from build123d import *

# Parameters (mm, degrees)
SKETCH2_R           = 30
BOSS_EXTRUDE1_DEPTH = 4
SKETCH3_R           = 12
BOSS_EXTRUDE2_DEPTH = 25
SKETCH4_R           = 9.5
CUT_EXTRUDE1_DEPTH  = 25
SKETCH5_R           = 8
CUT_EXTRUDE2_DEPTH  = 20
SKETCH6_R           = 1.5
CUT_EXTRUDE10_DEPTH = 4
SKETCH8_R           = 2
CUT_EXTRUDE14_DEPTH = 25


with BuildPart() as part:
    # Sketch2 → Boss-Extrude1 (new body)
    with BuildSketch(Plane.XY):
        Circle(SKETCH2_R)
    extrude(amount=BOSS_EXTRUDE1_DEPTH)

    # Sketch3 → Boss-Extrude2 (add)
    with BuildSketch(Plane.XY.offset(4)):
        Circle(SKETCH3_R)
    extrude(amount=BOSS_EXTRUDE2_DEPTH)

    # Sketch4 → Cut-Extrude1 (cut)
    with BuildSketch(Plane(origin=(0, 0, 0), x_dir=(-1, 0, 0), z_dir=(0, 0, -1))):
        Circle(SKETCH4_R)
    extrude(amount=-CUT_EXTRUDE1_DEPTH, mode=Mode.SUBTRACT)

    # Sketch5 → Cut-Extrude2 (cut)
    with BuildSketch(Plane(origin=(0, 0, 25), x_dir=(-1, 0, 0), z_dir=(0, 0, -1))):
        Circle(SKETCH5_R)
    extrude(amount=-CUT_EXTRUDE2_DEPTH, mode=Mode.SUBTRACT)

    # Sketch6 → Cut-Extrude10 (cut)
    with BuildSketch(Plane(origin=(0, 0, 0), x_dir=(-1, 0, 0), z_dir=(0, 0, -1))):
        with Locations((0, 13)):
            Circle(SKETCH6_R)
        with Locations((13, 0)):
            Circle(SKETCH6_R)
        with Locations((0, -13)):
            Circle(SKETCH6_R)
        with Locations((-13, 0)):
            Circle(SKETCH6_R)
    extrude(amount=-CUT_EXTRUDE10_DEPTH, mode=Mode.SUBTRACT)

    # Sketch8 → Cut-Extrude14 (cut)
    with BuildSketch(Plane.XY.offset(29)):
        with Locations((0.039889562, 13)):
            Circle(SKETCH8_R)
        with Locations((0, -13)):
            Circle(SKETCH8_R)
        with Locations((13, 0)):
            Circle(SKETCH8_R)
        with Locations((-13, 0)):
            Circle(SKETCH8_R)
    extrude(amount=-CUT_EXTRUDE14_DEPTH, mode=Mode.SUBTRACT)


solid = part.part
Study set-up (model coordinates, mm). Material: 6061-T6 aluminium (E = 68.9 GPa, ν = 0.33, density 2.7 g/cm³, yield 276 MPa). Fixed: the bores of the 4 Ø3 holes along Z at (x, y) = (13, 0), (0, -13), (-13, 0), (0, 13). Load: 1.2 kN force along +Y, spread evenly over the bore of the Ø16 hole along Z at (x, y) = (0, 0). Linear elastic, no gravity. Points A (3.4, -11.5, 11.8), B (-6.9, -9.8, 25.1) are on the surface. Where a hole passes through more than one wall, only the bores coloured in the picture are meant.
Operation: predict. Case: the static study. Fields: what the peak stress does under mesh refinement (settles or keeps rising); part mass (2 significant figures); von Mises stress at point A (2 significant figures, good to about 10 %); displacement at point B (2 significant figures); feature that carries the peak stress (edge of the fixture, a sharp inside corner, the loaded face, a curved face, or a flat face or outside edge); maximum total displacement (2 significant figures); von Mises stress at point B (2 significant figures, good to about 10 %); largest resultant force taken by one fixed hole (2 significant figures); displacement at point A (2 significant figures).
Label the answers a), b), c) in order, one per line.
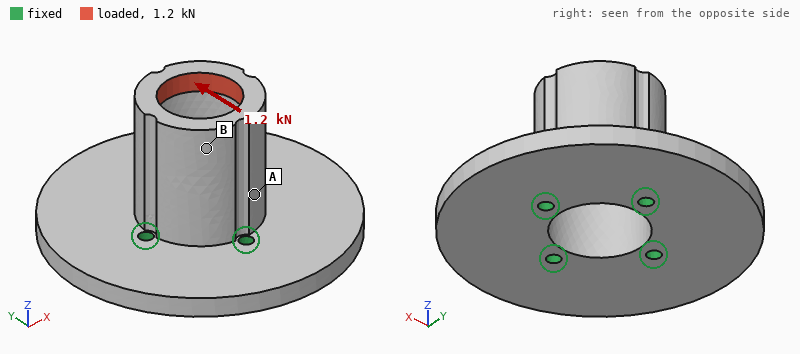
a) keeps rising
b) 39 g
c) 23 MPa
d) 29 µm
e) edge of the fixture
f) 36 µm
g) 8.4 MPa
h) 1.2 kN
i) 12 µm
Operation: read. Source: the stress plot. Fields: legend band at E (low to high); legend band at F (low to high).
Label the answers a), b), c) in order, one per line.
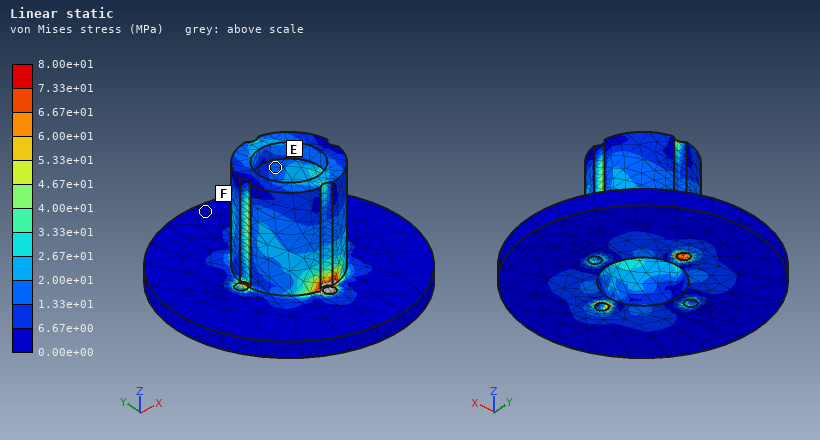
a) 1.33e+01 to 2.00e+01 MPa
b) 0.00e+00 to 6.67e+00 MPa
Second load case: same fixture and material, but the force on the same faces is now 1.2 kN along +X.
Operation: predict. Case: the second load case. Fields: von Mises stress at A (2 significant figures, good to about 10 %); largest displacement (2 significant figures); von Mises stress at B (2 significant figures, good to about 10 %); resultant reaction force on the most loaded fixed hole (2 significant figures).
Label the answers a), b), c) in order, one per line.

a) 18 MPa
b) 36 µm
c) 11 MPa
d) 1.2 kN
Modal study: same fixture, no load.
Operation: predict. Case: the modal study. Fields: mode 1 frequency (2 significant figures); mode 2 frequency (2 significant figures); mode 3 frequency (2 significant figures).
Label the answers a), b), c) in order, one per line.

a) 8400 Hz
b) 8700 Hz
c) 8700 Hz
